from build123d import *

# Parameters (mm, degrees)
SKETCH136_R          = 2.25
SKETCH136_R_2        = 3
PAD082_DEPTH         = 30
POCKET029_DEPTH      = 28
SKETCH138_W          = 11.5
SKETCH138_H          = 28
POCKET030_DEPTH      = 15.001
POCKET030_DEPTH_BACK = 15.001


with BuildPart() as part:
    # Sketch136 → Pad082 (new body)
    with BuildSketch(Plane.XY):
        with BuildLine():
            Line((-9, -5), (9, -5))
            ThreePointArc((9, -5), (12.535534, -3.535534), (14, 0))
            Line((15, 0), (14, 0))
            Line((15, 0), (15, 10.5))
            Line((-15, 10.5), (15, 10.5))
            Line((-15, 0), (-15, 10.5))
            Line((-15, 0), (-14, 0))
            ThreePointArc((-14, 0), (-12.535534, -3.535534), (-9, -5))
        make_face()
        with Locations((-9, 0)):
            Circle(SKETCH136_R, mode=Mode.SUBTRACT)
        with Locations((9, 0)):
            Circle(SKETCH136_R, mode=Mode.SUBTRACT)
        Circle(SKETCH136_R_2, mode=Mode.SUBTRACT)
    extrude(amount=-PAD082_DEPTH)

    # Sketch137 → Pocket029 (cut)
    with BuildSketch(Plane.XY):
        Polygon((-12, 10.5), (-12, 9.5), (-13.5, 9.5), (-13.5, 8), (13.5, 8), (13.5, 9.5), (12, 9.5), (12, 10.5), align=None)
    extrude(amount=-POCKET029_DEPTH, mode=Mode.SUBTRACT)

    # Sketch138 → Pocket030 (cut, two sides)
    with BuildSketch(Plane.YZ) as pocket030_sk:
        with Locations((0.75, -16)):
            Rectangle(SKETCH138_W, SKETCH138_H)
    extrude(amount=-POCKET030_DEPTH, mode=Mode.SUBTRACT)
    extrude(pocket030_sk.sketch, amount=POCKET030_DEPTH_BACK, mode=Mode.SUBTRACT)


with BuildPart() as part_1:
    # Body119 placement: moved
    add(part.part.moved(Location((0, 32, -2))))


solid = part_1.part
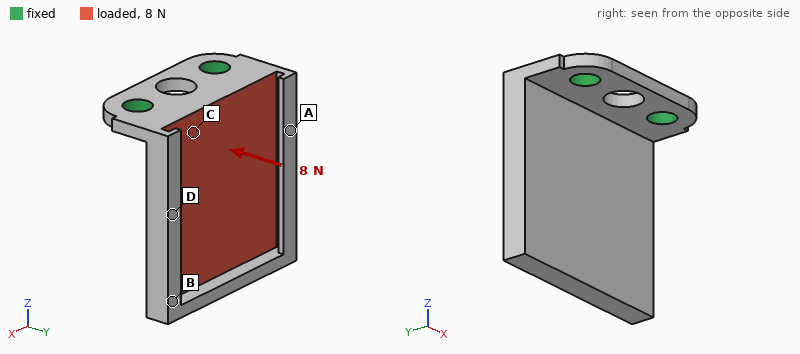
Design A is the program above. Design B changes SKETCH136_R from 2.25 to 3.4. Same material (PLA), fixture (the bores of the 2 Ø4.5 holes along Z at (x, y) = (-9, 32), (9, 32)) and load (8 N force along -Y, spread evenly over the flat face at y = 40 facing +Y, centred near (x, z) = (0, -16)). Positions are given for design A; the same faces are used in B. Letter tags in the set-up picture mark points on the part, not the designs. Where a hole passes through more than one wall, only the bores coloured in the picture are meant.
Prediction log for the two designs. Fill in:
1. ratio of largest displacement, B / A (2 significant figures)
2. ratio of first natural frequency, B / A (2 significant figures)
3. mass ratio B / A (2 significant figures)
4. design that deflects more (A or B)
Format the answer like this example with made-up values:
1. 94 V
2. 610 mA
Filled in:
1. 0.87
2. 1.1
3. 0.96
4. A
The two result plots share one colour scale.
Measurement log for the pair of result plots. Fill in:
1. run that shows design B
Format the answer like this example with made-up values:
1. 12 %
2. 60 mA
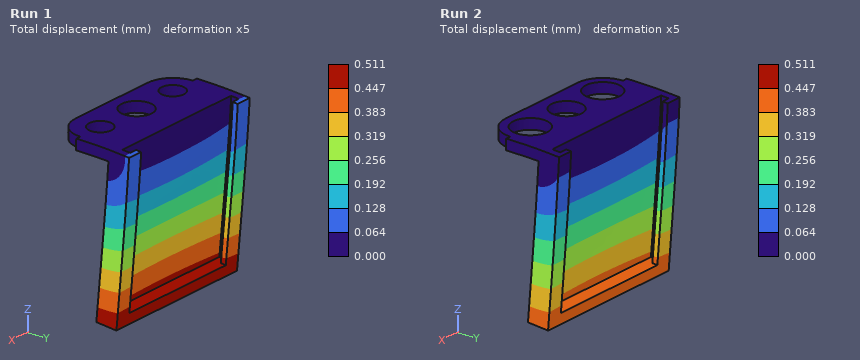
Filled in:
1. Run 2
